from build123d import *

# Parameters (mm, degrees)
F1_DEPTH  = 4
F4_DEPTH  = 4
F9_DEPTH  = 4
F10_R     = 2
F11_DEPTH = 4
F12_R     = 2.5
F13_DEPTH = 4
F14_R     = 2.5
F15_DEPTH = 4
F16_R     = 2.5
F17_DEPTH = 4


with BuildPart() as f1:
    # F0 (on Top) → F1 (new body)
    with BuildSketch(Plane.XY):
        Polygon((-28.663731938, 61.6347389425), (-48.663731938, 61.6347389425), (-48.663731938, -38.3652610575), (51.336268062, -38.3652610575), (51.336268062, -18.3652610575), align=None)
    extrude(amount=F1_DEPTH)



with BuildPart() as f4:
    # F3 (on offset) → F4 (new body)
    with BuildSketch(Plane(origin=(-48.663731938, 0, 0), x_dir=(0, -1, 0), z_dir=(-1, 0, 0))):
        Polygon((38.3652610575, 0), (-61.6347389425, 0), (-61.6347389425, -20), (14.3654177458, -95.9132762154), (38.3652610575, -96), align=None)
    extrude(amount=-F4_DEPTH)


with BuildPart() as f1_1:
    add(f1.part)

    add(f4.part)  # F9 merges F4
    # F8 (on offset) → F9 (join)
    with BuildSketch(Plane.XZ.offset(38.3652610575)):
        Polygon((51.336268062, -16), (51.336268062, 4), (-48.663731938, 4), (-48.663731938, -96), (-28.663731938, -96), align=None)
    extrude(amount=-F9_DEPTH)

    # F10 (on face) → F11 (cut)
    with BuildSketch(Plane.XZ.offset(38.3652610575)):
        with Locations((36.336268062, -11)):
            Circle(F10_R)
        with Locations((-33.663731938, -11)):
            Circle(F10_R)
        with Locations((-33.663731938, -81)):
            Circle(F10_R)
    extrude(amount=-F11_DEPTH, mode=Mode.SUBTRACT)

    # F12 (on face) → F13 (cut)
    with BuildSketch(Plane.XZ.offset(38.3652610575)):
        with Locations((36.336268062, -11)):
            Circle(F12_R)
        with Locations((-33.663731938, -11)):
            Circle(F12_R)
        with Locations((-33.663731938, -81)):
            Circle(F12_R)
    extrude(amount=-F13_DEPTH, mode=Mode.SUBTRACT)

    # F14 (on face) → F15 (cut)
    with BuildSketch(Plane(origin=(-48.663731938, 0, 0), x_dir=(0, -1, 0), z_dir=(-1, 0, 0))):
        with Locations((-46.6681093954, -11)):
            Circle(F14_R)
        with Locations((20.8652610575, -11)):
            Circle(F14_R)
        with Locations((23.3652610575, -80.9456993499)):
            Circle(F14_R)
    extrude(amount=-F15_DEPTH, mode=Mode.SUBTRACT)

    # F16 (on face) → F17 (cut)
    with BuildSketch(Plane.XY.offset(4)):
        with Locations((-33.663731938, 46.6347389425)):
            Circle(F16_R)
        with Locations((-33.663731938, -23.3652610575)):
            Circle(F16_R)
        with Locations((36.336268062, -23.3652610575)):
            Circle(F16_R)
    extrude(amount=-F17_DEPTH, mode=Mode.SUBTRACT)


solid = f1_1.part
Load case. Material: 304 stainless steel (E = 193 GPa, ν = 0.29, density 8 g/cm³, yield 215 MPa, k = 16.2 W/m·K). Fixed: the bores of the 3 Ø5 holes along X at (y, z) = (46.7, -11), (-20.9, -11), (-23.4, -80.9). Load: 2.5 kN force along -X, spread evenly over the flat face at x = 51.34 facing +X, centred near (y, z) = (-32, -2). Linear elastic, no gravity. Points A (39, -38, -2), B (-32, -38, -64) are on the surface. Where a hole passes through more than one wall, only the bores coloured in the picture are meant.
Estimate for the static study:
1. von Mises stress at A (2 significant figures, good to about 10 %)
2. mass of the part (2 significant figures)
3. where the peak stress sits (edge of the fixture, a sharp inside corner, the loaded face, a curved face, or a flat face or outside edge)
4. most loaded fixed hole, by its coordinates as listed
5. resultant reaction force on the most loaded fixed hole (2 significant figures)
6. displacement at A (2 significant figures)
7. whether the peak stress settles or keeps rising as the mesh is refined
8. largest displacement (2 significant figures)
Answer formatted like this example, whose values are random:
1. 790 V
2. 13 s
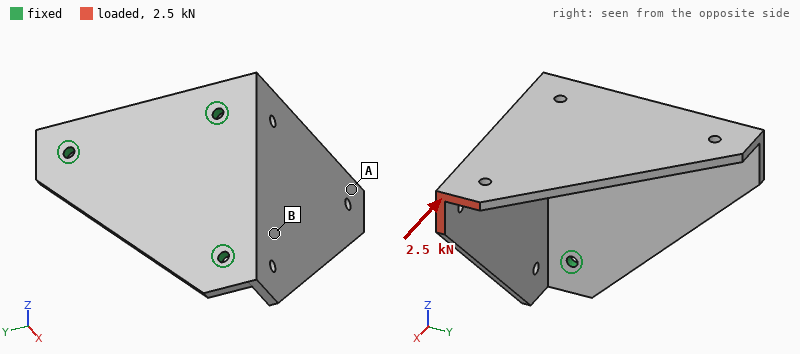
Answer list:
1. 20 MPa
2. 620 g
3. edge of the fixture
4. (-20.9, -11)
5. 3.0 kN
6. 71 µm
7. keeps rising
8. 82 µm
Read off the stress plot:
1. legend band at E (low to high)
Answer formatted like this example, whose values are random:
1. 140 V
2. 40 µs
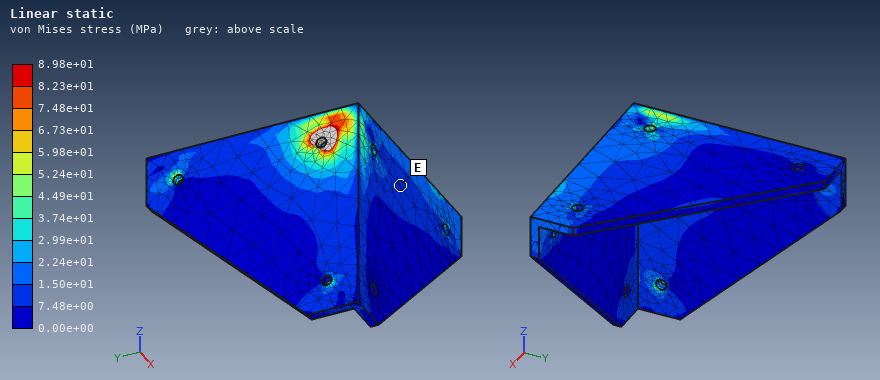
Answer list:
1. 7.48e+00 to 1.50e+01 MPa
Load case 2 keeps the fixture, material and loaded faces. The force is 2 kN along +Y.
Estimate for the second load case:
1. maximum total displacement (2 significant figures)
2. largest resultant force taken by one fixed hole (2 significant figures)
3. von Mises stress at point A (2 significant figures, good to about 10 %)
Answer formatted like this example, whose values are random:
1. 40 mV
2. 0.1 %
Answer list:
1. 0.29 mm
2. 3.1 kN
3. 84 MPa
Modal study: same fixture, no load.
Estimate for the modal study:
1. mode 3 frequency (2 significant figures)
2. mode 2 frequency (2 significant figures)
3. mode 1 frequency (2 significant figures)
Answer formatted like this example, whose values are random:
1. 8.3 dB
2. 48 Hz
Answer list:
1. 1800 Hz
2. 1600 Hz
3. 980 Hz
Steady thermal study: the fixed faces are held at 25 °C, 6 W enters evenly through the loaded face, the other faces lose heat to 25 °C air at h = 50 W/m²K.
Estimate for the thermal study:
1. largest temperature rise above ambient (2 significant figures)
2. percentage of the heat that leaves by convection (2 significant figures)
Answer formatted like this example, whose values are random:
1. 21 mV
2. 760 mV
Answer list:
1. 50 K
2. 98 %
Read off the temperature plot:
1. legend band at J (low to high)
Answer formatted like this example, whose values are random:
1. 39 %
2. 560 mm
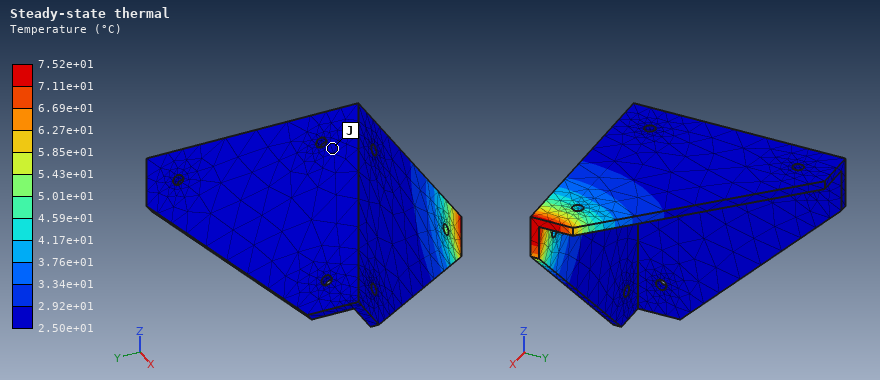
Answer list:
1. 2.50e+01 to 2.92e+01 °C
